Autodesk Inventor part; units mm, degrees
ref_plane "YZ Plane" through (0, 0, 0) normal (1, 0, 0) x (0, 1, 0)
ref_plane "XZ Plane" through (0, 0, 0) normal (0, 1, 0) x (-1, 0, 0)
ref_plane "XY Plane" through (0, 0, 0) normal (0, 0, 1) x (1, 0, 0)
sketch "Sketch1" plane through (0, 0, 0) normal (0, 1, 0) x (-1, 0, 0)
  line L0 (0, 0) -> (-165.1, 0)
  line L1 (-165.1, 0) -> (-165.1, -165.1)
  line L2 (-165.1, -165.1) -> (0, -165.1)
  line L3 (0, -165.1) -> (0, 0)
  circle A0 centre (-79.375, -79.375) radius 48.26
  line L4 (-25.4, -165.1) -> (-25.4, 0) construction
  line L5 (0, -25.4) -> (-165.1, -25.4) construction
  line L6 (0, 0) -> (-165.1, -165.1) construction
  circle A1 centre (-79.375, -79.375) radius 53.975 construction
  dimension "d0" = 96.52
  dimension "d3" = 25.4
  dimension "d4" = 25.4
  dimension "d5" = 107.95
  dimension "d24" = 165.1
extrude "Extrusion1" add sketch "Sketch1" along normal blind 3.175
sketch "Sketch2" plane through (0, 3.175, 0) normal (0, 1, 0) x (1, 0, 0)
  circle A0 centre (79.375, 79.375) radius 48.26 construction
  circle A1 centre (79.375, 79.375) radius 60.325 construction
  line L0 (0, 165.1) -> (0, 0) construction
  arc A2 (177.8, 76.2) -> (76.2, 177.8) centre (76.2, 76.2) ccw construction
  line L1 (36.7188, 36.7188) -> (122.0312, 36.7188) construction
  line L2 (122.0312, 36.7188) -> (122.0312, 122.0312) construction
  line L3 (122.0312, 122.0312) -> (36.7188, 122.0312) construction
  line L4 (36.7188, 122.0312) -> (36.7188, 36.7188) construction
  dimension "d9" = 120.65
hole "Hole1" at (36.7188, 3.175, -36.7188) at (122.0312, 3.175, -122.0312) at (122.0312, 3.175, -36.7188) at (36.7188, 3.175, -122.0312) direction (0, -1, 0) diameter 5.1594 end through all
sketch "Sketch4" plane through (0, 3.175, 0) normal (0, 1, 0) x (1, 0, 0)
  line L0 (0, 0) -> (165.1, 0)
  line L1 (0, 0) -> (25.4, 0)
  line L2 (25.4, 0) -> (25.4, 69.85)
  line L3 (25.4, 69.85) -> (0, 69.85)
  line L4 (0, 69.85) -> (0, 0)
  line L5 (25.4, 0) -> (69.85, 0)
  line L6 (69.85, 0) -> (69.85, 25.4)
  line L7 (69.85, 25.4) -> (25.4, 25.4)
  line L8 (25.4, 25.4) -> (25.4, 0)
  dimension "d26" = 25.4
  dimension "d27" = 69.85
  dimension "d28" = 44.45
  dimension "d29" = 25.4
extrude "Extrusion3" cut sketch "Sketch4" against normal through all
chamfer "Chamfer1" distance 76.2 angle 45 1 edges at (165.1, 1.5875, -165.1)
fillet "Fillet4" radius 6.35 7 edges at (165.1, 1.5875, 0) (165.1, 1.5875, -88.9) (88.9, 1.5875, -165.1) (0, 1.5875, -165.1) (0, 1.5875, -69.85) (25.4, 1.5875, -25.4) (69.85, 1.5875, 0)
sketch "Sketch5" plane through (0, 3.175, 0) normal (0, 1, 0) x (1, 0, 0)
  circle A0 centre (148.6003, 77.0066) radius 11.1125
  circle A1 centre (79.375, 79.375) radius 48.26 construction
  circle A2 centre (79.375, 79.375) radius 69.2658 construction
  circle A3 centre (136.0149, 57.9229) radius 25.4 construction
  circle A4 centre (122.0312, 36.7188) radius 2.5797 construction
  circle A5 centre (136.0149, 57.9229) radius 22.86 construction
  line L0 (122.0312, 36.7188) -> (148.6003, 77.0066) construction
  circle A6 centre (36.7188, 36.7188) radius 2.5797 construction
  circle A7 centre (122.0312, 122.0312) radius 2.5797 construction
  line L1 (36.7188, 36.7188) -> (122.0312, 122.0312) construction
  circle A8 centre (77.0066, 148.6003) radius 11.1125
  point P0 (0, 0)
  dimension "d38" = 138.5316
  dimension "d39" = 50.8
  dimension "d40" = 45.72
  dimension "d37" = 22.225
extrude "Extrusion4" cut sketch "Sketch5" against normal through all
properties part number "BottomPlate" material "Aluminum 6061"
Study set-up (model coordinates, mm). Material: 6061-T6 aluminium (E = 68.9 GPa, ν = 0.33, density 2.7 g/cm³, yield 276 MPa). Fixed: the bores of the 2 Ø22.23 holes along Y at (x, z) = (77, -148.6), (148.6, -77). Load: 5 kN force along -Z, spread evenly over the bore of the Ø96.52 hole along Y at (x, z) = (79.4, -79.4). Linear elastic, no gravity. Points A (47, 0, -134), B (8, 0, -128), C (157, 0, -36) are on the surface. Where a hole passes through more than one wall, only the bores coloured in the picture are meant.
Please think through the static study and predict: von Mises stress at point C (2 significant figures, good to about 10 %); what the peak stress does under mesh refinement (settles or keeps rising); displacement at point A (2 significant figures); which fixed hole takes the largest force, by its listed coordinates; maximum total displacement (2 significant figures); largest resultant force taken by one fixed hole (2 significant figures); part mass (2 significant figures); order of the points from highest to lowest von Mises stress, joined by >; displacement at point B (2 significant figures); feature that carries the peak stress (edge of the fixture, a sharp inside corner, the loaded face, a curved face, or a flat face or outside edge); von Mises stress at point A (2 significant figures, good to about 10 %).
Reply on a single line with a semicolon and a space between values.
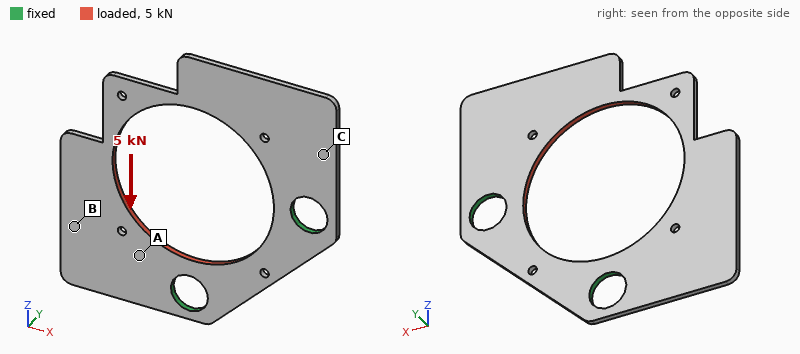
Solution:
19 MPa; keeps rising; 0.047 mm; (77, -148.6); 0.22 mm; 2.8 kN; 110 g; A > C > B; 0.13 mm; edge of the fixture; 36 MPa
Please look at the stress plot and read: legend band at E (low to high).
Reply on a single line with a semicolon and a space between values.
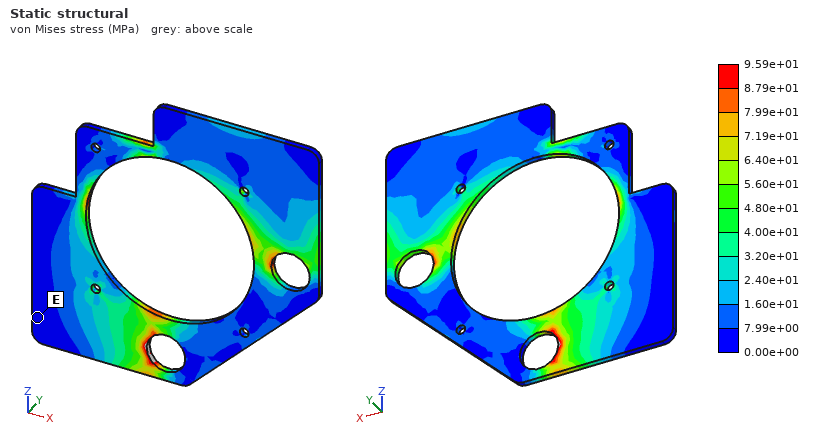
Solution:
0.00e+00 to 7.99e+00 MPa
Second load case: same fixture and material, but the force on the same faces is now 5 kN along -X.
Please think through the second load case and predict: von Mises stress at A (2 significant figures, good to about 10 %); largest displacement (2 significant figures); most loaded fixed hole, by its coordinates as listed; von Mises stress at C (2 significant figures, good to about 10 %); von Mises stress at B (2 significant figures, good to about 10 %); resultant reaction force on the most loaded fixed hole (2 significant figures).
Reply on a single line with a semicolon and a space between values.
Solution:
21 MPa; 0.22 mm; (148.6, -77); 18 MPa; 12 MPa; 2.8 kN
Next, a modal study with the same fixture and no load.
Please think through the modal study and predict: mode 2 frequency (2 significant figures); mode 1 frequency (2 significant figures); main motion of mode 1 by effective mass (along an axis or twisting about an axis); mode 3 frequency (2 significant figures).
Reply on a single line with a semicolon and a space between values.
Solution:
380 Hz; 250 Hz; along Y; 620 Hz
